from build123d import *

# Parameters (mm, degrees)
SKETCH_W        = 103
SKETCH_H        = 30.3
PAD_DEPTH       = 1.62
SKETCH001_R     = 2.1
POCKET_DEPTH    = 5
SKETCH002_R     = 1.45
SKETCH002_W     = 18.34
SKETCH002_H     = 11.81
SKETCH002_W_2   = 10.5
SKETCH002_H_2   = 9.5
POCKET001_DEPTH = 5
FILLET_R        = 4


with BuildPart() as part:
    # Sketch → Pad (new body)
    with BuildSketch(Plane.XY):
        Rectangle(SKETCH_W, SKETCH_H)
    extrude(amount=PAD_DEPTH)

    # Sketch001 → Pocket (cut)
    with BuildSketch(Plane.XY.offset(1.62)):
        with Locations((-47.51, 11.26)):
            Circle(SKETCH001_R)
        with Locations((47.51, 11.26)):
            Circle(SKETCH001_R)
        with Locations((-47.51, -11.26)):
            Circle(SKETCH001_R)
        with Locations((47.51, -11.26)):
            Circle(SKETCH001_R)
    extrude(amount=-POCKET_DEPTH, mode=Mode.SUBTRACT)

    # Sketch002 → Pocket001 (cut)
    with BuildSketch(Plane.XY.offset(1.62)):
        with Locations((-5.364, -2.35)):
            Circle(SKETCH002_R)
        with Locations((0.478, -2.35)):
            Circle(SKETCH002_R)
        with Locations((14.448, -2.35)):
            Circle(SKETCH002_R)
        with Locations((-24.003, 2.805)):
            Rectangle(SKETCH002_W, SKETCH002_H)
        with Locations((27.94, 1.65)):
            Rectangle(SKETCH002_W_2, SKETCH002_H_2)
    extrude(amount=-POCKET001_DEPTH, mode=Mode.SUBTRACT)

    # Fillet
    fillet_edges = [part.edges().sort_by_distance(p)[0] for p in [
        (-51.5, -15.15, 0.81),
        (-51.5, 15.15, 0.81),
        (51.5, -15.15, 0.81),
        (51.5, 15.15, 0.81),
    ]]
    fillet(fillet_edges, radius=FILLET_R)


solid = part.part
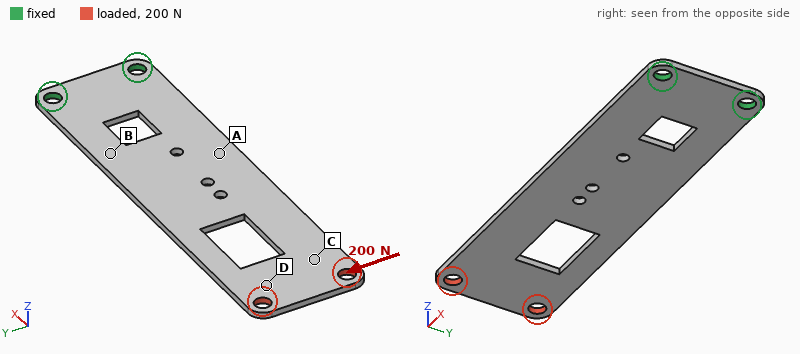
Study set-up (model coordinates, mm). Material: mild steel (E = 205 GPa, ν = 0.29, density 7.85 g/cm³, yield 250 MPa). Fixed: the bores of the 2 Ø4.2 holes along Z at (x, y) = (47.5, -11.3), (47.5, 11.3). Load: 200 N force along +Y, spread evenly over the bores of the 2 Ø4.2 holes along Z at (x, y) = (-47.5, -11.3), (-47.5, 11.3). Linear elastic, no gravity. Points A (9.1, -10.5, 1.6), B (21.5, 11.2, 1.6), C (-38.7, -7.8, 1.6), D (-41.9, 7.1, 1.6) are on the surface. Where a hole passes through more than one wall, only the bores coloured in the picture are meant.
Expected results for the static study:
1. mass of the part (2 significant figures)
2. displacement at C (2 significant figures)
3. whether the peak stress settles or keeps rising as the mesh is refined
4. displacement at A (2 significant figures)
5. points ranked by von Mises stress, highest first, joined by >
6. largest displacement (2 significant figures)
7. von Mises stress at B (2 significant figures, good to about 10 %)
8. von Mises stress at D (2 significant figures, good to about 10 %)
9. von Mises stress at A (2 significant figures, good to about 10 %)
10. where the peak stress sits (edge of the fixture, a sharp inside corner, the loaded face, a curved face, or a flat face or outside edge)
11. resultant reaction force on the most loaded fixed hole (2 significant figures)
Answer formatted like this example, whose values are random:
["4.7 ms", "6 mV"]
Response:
["35 g", "80 µm", "keeps rising", "22 µm", "B > A > D > C", "97 µm", "43 MPa", "17 MPa", "31 MPa", "edge of the fixture", "810 N"]
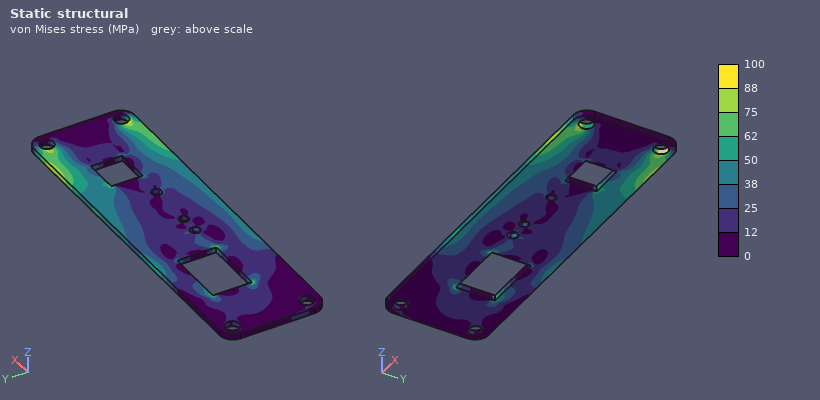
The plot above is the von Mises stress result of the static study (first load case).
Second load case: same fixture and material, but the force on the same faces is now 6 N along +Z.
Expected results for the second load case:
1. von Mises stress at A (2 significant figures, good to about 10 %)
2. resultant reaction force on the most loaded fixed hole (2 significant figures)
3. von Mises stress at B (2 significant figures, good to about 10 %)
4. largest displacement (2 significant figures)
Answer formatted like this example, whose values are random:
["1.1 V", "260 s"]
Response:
["27 MPa", "3.0 N", "42 MPa", "0.97 mm"]
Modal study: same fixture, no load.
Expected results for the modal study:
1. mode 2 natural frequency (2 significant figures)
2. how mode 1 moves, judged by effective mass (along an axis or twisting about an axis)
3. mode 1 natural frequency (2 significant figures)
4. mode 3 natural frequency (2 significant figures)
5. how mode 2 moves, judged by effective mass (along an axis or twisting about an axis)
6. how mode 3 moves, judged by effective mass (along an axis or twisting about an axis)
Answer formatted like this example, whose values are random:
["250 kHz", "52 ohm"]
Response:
["830 Hz", "along Z", "140 Hz", "890 Hz", "along Z", "twisting about X"]
